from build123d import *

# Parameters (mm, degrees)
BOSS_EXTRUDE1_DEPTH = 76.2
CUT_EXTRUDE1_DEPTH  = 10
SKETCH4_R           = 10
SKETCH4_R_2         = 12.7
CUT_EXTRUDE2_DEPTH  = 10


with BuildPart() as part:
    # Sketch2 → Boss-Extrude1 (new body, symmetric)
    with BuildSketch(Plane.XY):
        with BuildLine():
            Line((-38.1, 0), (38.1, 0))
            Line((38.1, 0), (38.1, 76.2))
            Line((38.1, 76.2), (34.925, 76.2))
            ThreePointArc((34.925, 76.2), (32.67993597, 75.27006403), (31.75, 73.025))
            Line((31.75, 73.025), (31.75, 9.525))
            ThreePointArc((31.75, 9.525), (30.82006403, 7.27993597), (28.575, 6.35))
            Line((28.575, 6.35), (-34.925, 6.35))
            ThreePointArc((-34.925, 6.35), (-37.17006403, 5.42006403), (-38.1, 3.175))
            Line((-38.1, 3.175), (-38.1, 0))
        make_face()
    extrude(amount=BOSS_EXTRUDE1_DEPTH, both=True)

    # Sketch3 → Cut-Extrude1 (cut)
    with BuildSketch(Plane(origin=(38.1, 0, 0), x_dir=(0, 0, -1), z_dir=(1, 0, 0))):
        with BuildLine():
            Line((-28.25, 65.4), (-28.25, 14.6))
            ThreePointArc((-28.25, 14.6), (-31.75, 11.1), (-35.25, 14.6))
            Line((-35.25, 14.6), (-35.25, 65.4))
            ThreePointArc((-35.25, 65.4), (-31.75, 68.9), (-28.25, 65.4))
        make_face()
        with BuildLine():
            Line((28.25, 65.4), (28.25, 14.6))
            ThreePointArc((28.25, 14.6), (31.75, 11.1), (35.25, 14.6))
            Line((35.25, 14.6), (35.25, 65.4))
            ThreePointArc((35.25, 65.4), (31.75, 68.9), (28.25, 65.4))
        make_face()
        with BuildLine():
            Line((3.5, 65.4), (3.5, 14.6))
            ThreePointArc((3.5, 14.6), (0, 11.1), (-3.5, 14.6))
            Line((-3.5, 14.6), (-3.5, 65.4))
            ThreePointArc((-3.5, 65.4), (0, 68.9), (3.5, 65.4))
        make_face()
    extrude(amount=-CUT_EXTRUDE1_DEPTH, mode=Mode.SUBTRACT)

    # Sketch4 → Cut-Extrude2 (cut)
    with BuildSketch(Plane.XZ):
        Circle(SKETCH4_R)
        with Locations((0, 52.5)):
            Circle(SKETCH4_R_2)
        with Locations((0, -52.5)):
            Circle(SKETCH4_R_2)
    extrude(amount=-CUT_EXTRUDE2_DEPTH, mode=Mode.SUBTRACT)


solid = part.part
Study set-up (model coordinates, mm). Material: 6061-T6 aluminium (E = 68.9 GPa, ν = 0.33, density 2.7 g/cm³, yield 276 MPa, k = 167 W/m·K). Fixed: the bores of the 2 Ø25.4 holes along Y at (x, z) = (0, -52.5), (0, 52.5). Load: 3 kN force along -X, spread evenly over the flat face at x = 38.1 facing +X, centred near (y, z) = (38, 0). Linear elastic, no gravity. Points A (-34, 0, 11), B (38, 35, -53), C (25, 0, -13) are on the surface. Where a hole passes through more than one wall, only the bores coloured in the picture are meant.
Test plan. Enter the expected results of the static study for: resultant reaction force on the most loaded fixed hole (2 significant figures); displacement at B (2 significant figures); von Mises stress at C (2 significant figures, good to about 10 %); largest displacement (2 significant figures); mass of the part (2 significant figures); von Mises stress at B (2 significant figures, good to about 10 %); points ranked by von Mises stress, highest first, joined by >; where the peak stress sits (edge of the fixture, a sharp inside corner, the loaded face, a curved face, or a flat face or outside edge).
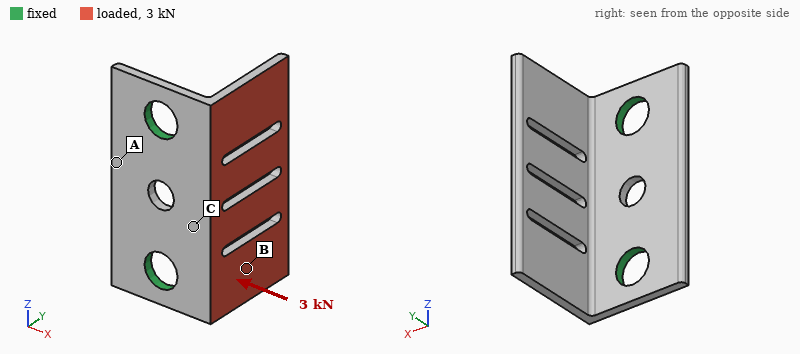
1.5 kN
0.55 mm
71 MPa
1.4 mm
340 g
36 MPa
C > B > A
a flat face or outside edge
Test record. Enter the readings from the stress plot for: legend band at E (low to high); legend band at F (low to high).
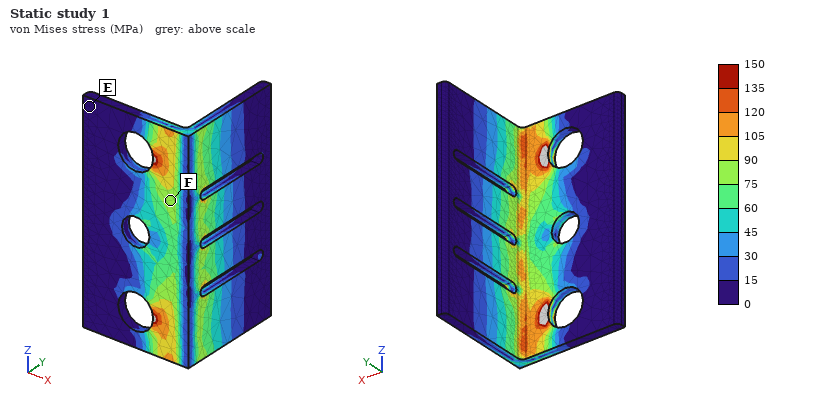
0 to 15 MPa
75 to 90 MPa
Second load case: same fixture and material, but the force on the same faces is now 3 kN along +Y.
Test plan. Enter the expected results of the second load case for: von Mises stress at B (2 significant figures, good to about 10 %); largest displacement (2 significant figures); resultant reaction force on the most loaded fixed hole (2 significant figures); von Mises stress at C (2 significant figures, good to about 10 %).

7.2 MPa
0.52 mm
1.5 kN
23 MPa
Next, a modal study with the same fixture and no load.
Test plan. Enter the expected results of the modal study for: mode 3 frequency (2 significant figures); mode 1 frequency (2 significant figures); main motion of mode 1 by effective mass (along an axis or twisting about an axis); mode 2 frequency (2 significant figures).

2200 Hz
670 Hz
along X
1100 Hz
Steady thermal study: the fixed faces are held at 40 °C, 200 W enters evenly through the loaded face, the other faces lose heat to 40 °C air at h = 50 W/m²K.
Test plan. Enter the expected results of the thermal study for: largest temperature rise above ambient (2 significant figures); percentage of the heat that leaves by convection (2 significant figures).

67 K
24 %
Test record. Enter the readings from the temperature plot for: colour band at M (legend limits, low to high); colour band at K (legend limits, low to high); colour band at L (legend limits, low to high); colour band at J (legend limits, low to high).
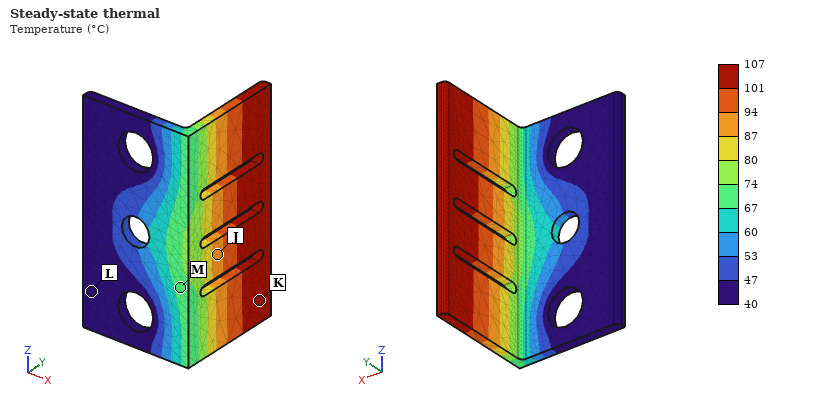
67 to 74 °C
101 to 107 °C
40 to 47 °C
87 to 94 °C
